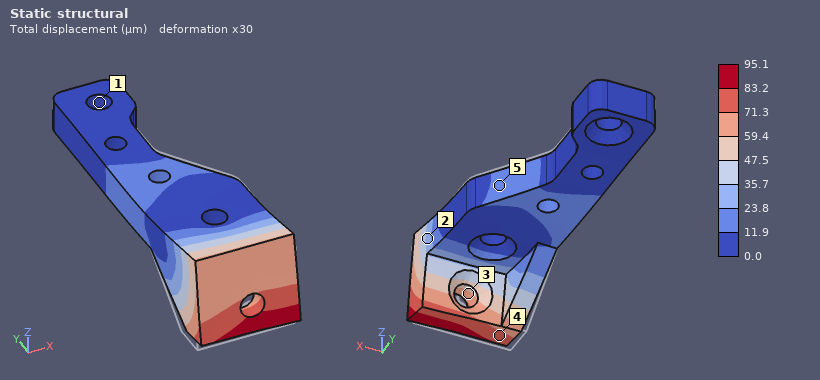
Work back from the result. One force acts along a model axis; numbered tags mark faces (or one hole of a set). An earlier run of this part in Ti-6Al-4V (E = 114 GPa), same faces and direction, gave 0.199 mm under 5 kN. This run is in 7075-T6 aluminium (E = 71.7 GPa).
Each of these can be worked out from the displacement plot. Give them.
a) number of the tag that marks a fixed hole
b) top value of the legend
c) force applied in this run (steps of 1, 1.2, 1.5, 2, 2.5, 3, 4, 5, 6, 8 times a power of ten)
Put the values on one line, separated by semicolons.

1; 95.1 µm; 1.5 kN
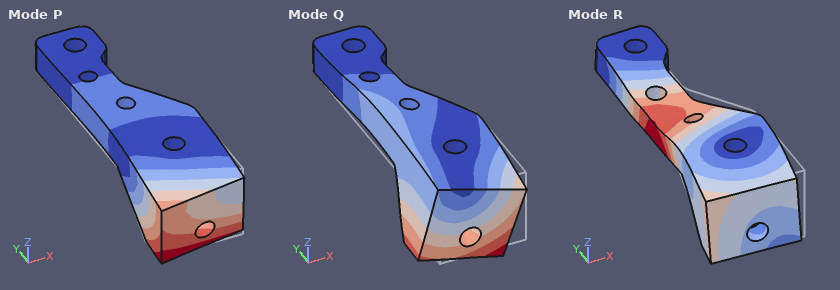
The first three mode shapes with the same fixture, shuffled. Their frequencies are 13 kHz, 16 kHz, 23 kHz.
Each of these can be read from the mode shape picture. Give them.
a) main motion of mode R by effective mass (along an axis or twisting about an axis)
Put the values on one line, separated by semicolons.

along Z
